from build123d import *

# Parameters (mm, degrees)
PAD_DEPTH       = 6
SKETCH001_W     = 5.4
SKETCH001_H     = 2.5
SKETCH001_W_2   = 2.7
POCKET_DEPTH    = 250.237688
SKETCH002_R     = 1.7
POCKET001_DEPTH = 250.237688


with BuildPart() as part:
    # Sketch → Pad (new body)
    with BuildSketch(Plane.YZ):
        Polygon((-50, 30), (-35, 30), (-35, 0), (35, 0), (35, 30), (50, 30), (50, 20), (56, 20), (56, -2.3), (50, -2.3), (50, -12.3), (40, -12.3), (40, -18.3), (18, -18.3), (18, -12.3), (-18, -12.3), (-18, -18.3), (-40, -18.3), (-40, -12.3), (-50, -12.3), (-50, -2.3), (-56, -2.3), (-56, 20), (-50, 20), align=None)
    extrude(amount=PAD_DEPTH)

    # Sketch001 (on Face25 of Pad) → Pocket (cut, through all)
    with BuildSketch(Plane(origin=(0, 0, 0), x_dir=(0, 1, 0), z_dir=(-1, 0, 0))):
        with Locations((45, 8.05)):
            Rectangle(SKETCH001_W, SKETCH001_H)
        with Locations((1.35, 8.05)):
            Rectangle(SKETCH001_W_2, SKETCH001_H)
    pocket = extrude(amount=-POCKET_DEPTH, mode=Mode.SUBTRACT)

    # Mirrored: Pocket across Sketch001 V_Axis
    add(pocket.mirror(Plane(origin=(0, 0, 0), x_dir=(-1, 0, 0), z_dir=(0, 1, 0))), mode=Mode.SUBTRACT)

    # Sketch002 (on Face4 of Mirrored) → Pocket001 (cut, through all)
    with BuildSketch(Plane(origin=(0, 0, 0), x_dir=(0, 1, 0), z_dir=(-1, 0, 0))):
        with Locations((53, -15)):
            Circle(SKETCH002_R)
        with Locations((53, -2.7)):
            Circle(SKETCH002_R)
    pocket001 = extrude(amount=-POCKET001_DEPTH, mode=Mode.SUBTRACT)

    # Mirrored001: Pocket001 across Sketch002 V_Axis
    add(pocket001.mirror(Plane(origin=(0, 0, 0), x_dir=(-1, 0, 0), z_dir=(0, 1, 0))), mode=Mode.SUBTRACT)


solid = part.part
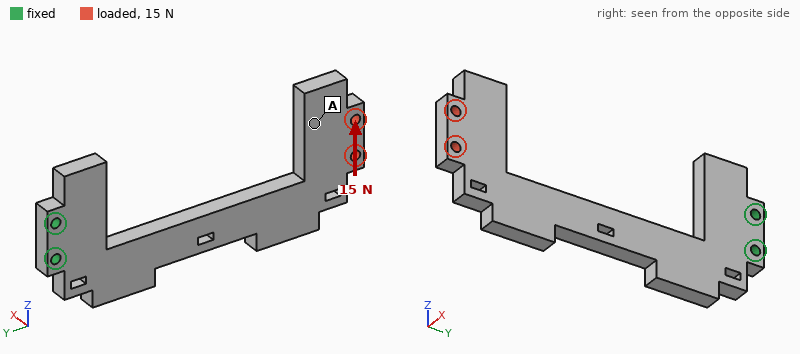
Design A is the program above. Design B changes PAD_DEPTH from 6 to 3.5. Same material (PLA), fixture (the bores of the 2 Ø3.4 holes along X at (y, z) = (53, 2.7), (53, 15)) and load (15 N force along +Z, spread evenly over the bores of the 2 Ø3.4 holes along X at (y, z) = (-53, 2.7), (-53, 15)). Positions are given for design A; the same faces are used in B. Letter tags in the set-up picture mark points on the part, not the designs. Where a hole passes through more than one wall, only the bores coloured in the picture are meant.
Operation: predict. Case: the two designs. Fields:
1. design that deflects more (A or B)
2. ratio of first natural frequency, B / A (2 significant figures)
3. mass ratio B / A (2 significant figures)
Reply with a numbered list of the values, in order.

1. B
2. 0.60
3. 0.58
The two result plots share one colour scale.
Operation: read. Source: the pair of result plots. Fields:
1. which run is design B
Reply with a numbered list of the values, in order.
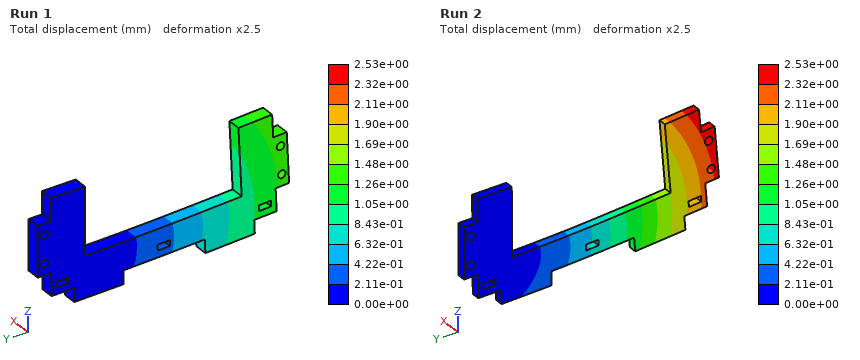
1. Run 2
